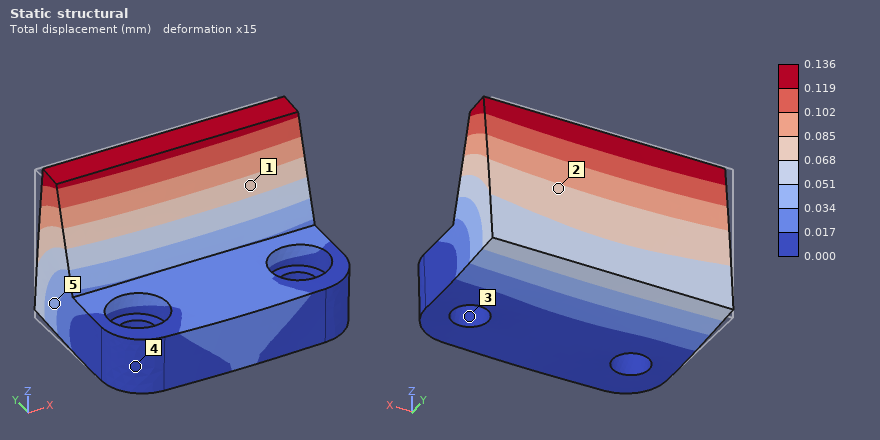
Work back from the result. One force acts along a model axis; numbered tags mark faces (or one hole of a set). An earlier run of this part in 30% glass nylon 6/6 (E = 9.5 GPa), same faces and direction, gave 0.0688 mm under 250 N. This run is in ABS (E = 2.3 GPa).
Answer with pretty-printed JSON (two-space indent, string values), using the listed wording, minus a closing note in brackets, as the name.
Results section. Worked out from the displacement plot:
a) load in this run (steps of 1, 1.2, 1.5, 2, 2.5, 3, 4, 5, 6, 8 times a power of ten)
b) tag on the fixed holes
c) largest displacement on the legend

{
  "load in this run": "120 N",
  "tag on the fixed holes": "3",
  "largest displacement on the legend": "0.136 mm"
}
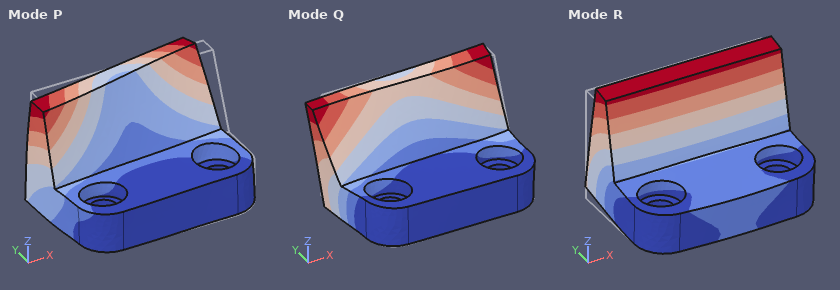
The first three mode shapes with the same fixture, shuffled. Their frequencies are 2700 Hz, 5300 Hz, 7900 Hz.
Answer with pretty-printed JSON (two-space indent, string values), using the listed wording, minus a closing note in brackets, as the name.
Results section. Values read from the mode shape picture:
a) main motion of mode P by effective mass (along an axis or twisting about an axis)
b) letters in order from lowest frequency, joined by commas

{
  "main motion of mode P by effective mass": "along X",
  "letters in order from lowest frequency, joined by commas": "R, Q, P"
}
